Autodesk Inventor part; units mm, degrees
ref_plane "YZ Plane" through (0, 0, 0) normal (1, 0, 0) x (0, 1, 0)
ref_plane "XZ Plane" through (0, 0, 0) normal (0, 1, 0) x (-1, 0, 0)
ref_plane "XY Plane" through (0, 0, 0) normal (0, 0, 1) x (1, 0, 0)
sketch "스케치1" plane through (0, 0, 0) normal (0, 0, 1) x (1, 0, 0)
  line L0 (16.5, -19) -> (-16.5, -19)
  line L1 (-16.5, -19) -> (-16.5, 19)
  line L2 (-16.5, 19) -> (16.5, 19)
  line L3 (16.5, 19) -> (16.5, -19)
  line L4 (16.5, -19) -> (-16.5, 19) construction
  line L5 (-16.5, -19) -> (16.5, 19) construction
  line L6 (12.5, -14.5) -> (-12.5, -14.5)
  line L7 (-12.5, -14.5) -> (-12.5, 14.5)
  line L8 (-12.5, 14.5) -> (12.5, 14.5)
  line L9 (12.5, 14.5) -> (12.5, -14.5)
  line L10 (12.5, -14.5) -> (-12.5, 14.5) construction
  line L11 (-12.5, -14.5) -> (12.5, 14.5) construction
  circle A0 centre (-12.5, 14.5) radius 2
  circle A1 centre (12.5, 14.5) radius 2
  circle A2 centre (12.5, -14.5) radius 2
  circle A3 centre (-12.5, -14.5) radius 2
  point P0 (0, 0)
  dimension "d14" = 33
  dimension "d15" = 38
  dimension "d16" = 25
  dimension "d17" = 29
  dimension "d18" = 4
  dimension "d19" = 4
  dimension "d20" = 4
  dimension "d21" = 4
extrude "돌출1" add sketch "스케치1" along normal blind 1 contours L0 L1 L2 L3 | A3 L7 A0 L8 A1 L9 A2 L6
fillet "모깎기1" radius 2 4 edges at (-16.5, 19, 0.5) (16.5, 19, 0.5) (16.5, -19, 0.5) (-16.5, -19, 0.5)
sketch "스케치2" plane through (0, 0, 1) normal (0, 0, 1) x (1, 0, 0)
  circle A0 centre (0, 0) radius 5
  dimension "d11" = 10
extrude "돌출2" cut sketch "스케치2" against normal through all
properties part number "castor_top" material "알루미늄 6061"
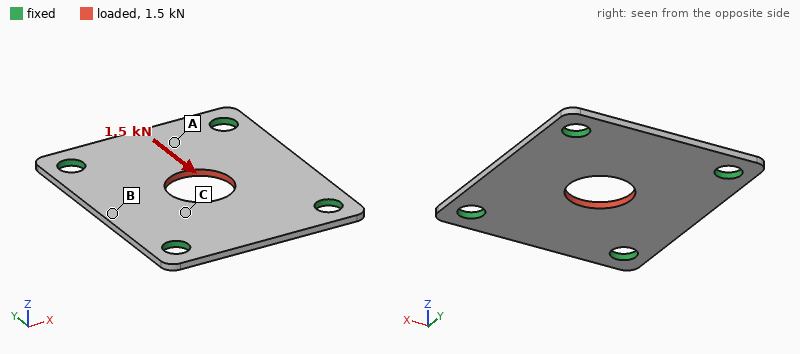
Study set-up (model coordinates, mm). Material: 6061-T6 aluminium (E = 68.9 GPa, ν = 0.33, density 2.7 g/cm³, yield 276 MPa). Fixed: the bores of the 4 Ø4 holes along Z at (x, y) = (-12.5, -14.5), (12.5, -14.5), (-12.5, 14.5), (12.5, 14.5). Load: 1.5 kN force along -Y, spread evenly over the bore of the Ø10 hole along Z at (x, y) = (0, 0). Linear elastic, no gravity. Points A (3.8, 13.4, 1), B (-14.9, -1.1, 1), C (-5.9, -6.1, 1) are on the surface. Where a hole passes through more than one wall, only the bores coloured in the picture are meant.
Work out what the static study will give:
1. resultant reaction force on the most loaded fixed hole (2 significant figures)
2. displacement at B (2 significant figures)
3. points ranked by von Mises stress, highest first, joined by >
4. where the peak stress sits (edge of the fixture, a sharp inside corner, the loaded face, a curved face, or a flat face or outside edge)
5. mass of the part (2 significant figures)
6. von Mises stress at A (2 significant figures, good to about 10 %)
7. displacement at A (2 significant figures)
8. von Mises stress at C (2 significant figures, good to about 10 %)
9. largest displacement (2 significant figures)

410 N
2.5 µm
C > A > B
edge of the fixture
3.0 g
23 MPa
6.9 µm
41 MPa
11 µm
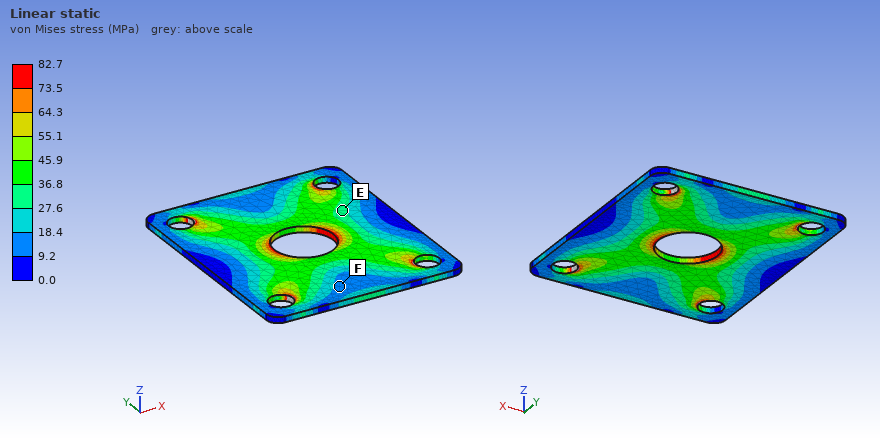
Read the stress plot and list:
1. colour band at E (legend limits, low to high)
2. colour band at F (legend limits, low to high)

27.6 to 36.8 MPa
9.2 to 18.4 MPa
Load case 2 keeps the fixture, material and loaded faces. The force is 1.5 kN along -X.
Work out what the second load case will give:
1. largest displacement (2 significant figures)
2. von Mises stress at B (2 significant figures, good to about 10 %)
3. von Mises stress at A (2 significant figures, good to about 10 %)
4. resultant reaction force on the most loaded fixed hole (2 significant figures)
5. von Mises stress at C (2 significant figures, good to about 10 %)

15 µm
25 MPa
26 MPa
430 N
45 MPa
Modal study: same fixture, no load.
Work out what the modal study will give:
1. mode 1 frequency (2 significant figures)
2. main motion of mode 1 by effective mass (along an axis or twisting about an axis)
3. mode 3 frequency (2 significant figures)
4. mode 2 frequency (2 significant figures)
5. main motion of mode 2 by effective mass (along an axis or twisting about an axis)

6200 Hz
along Z
9800 Hz
8400 Hz
twisting about Y
